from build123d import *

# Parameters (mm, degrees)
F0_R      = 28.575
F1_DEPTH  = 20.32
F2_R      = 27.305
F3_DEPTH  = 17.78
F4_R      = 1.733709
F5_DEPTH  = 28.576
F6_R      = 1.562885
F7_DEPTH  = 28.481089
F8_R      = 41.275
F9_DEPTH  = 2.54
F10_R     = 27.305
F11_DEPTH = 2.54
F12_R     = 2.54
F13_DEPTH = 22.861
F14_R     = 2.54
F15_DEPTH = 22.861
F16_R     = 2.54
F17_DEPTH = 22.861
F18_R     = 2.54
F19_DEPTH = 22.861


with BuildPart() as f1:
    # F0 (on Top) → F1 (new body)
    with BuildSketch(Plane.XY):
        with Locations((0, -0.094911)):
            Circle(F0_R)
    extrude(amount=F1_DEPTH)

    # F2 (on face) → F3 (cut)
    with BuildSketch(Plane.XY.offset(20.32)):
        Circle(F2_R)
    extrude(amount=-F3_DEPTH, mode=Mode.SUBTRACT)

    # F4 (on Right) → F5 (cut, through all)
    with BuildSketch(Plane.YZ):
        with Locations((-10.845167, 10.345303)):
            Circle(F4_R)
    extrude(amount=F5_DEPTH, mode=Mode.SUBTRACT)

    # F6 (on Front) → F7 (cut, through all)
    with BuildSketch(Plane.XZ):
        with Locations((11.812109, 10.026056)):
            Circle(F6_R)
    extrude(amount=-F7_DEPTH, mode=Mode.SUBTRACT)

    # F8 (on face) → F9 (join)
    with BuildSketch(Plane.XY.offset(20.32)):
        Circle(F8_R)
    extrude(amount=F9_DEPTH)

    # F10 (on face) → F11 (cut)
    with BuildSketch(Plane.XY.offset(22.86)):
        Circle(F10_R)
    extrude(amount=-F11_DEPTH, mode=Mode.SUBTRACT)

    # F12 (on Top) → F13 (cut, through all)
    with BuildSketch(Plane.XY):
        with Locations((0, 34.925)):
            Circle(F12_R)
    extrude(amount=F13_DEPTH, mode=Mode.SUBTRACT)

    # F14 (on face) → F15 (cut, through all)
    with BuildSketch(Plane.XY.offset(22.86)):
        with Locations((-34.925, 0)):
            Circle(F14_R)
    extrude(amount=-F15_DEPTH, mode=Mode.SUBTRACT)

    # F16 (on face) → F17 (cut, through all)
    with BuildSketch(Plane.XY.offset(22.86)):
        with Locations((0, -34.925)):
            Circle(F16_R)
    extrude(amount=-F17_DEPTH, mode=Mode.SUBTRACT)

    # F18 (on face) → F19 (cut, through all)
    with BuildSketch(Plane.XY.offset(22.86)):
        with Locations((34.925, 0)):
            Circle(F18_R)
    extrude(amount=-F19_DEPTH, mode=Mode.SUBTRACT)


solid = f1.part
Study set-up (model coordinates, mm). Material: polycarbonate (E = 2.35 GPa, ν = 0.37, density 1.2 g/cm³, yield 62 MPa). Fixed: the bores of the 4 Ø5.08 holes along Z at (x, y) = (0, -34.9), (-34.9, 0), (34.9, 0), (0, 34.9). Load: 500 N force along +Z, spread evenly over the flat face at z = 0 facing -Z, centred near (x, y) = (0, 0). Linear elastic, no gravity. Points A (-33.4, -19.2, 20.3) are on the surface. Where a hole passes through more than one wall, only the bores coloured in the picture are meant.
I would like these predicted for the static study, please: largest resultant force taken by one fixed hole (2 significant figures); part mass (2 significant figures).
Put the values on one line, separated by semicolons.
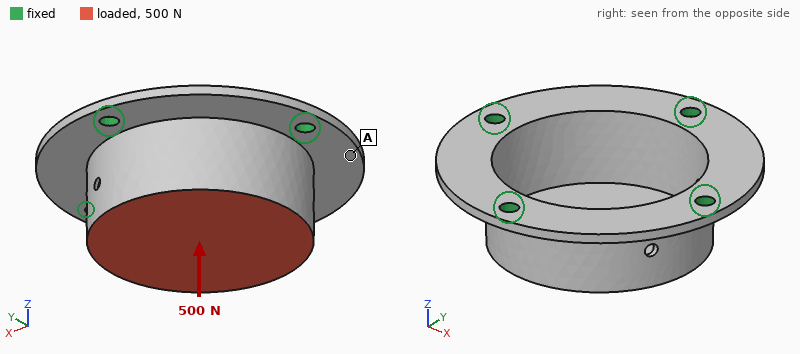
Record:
130 N; 21 g
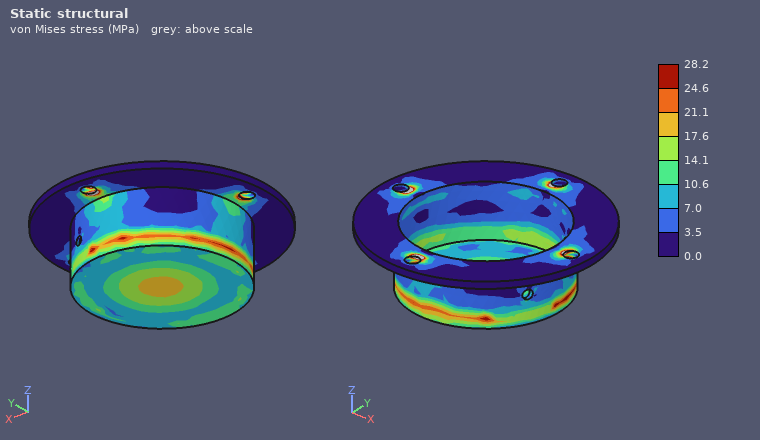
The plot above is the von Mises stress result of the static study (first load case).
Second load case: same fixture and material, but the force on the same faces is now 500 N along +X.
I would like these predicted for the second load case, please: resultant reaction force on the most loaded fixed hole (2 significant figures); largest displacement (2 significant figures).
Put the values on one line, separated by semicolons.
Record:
200 N; 0.36 mm
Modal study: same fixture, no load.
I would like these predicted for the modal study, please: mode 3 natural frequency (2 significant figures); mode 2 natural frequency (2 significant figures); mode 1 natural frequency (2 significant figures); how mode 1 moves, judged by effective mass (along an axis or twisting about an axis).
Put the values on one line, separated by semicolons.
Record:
1700 Hz; 1700 Hz; 1400 Hz; along Z
